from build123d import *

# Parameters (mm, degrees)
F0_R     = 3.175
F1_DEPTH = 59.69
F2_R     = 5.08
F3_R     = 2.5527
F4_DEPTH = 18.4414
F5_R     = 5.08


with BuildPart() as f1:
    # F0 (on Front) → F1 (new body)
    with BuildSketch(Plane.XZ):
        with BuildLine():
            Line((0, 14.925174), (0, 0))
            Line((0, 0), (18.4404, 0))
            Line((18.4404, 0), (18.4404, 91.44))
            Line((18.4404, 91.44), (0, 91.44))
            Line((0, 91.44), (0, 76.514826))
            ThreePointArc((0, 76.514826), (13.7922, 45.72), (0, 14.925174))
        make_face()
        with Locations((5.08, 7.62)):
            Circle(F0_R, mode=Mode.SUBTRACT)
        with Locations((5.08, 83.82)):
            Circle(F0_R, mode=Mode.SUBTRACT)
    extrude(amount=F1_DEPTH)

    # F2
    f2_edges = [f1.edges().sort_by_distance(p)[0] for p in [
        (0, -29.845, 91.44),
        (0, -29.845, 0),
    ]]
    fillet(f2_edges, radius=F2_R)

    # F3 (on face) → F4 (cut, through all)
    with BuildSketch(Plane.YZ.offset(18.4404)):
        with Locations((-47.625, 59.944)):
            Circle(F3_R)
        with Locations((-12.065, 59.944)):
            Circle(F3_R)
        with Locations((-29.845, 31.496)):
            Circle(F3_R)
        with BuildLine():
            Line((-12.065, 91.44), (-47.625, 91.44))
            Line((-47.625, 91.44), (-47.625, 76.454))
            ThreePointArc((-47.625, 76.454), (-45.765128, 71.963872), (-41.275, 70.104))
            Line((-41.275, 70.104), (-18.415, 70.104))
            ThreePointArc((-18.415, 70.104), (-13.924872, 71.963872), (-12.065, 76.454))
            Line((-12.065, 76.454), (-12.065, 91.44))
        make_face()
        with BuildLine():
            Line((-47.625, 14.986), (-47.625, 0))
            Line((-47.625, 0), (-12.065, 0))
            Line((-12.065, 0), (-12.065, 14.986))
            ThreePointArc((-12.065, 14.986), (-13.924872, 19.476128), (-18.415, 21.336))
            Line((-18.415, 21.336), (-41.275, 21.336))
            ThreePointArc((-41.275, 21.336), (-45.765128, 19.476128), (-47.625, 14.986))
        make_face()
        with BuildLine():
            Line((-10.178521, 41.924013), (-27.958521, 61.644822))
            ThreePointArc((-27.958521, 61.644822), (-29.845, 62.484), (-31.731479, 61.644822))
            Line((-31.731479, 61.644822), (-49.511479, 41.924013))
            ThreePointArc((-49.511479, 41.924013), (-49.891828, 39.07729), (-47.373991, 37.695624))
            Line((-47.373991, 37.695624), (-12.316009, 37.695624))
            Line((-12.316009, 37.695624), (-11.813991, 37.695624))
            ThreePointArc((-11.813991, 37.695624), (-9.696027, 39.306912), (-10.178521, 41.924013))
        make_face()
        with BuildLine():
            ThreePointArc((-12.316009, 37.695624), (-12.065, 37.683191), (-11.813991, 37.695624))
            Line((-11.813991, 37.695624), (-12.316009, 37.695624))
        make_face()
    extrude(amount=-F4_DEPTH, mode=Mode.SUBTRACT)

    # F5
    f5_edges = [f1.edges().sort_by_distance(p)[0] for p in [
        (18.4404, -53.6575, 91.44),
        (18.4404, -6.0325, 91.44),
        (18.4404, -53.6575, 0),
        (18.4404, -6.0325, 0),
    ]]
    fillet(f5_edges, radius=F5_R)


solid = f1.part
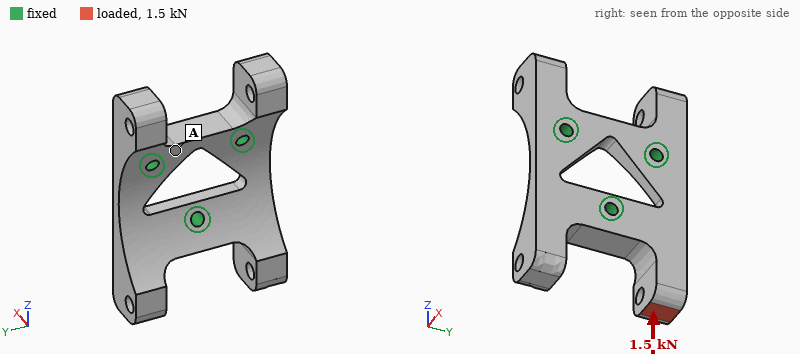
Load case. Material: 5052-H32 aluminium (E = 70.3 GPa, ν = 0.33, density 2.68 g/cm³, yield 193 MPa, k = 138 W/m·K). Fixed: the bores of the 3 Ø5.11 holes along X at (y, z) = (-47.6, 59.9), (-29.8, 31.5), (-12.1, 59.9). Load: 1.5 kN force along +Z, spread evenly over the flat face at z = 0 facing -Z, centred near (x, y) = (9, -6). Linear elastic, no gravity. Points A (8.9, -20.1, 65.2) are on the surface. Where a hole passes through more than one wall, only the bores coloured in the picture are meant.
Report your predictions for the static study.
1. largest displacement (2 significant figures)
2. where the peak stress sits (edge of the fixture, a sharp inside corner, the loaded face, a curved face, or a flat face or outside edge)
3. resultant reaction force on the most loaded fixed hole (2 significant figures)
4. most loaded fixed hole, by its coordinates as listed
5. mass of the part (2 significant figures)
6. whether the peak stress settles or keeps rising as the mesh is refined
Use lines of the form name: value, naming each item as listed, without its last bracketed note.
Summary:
largest displacement: 0.11 mm
where the peak stress sits: edge of the fixture
resultant reaction force on the most loaded fixed hole: 1.2 kN
most loaded fixed hole, by its coordinates as listed: (-12.1, 59.9)
mass of the part: 91 g
whether the peak stress settles or keeps rising as the mesh is refined: keeps rising
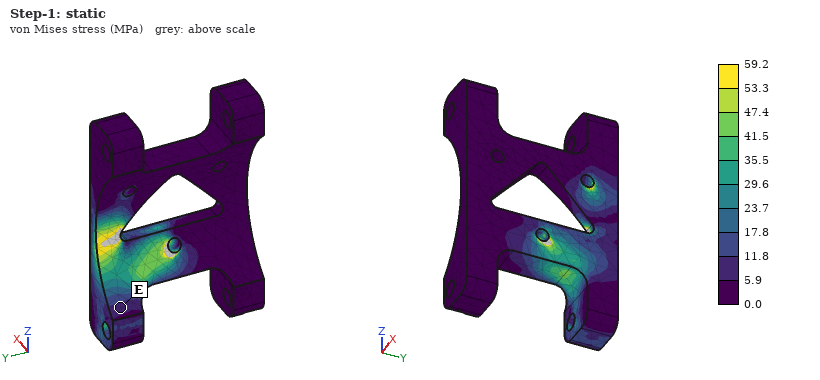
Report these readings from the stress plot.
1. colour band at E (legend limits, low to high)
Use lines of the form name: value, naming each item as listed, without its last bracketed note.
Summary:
colour band at E: 5.9 to 11.8 MPa
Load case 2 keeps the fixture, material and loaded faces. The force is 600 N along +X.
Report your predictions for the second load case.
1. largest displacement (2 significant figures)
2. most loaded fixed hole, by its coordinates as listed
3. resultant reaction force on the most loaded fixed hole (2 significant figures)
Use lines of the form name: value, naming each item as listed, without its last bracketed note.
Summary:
largest displacement: 0.25 mm
most loaded fixed hole, by its coordinates as listed: (-29.8, 31.5)
resultant reaction force on the most loaded fixed hole: 790 N
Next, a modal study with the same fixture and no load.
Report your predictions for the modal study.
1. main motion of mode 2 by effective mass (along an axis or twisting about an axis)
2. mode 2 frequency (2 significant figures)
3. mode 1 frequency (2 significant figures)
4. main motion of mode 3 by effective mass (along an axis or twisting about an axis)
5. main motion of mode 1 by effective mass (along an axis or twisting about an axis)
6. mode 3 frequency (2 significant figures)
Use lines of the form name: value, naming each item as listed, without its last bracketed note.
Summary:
main motion of mode 2 by effective mass: along X
mode 2 frequency: 3400 Hz
mode 1 frequency: 3000 Hz
main motion of mode 3 by effective mass: along X
main motion of mode 1 by effective mass: twisting about Z
mode 3 frequency: 6000 Hz
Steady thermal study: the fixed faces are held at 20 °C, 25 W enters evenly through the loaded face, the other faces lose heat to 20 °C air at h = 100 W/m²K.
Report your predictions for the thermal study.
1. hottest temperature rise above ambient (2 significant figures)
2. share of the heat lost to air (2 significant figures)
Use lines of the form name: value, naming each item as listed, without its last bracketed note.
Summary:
hottest temperature rise above ambient: 43 K
share of the heat lost to air: 27 %
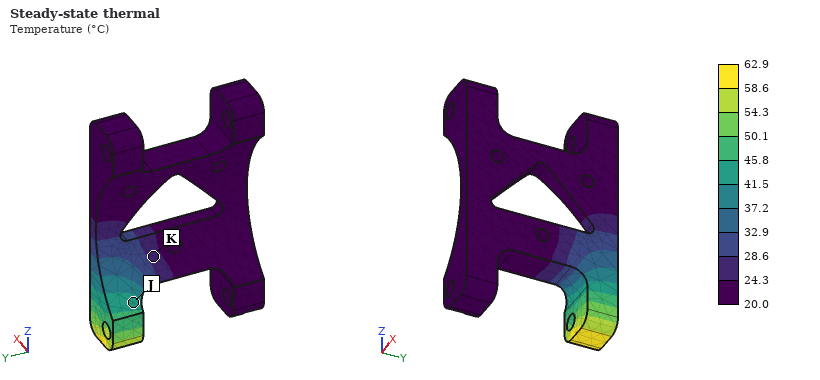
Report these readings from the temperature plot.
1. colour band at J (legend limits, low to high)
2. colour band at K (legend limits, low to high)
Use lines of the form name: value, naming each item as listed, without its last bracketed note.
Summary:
colour band at J: 41.5 to 45.8 °C
colour band at K: 24.3 to 28.6 °C
